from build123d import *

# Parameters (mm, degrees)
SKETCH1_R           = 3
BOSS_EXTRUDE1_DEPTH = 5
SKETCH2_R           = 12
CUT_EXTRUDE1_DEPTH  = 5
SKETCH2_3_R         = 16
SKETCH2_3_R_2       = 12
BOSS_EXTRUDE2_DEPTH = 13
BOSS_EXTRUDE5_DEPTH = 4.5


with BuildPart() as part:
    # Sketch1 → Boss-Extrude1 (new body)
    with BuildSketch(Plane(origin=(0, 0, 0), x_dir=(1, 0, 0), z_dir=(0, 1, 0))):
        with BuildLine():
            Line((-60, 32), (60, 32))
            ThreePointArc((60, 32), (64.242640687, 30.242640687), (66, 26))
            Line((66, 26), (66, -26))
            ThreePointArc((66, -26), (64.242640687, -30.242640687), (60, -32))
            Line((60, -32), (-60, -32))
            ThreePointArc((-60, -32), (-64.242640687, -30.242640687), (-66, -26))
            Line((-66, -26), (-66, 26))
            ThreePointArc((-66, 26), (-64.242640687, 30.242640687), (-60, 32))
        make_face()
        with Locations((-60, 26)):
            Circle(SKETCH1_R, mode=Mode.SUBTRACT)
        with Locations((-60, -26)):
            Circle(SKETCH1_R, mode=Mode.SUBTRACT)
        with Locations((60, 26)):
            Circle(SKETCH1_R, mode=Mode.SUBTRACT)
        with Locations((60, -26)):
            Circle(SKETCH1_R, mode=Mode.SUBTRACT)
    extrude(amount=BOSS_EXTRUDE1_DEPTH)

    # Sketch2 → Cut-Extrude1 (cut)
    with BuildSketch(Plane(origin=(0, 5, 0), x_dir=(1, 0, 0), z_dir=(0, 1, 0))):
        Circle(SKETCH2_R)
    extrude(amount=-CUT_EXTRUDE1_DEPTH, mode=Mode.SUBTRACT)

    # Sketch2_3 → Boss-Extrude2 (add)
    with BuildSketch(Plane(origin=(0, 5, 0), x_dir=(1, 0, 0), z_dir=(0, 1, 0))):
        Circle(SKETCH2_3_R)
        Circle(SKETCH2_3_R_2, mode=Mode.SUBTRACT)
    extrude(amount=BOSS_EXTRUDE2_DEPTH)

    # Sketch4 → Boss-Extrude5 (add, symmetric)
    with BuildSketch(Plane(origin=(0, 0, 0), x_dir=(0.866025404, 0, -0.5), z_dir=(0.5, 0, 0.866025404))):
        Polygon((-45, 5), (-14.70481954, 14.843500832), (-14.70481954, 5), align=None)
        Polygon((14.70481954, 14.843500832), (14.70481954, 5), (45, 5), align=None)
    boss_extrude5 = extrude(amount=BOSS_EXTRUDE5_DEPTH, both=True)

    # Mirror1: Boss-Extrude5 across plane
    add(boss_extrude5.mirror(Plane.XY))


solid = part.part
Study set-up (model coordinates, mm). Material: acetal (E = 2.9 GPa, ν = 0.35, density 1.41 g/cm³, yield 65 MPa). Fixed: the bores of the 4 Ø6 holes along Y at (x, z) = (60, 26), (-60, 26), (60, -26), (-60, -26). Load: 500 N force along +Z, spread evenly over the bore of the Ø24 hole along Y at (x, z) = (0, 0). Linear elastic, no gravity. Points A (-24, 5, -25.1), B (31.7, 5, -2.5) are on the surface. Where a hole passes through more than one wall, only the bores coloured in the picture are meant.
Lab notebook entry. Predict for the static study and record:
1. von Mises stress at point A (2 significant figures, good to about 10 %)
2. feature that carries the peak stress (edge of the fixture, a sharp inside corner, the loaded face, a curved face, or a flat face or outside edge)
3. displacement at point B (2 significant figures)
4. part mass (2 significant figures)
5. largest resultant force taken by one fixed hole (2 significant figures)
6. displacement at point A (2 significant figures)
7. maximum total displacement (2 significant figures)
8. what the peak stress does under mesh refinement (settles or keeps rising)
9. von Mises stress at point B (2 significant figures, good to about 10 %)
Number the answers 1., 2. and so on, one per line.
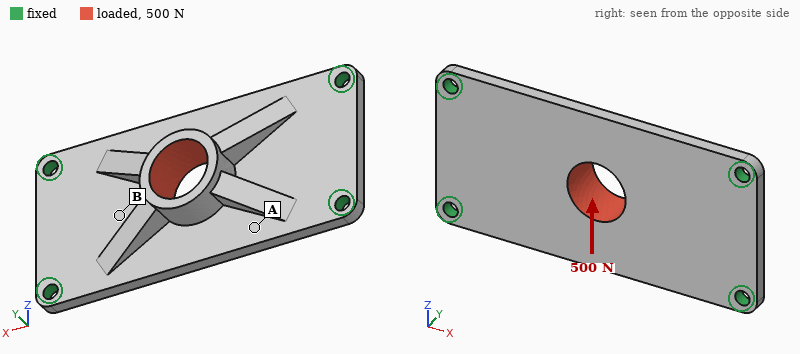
1. 1.7 MPa
2. edge of the fixture
3. 0.042 mm
4. 69 g
5. 200 N
6. 0.15 mm
7. 0.23 mm
8. keeps rising
9. 3.0 MPa
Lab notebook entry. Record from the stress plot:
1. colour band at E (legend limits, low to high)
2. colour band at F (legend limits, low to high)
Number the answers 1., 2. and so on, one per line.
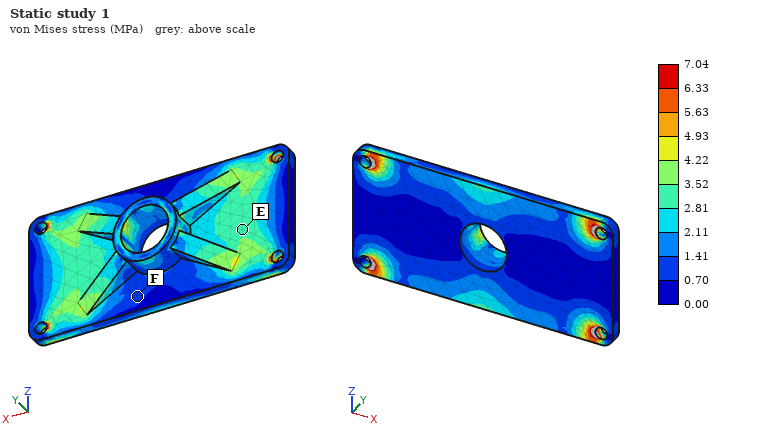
1. 2.81 to 3.52 MPa
2. 0.70 to 1.41 MPa
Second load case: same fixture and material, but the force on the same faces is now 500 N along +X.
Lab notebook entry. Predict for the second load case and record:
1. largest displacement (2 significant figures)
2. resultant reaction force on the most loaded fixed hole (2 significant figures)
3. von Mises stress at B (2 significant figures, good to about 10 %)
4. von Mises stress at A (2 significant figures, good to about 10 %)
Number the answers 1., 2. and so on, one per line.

1. 52 µm
2. 130 N
3. 1.4 MPa
4. 0.99 MPa
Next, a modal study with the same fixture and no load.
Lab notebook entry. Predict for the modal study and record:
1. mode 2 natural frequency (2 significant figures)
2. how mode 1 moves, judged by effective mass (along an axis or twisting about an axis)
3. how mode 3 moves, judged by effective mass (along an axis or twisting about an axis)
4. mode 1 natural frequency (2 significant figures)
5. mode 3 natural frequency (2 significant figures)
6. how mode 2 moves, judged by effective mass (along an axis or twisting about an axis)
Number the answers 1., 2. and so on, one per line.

1. 940 Hz
2. along Y
3. twisting about Z
4. 600 Hz
5. 1500 Hz
6. twisting about X
